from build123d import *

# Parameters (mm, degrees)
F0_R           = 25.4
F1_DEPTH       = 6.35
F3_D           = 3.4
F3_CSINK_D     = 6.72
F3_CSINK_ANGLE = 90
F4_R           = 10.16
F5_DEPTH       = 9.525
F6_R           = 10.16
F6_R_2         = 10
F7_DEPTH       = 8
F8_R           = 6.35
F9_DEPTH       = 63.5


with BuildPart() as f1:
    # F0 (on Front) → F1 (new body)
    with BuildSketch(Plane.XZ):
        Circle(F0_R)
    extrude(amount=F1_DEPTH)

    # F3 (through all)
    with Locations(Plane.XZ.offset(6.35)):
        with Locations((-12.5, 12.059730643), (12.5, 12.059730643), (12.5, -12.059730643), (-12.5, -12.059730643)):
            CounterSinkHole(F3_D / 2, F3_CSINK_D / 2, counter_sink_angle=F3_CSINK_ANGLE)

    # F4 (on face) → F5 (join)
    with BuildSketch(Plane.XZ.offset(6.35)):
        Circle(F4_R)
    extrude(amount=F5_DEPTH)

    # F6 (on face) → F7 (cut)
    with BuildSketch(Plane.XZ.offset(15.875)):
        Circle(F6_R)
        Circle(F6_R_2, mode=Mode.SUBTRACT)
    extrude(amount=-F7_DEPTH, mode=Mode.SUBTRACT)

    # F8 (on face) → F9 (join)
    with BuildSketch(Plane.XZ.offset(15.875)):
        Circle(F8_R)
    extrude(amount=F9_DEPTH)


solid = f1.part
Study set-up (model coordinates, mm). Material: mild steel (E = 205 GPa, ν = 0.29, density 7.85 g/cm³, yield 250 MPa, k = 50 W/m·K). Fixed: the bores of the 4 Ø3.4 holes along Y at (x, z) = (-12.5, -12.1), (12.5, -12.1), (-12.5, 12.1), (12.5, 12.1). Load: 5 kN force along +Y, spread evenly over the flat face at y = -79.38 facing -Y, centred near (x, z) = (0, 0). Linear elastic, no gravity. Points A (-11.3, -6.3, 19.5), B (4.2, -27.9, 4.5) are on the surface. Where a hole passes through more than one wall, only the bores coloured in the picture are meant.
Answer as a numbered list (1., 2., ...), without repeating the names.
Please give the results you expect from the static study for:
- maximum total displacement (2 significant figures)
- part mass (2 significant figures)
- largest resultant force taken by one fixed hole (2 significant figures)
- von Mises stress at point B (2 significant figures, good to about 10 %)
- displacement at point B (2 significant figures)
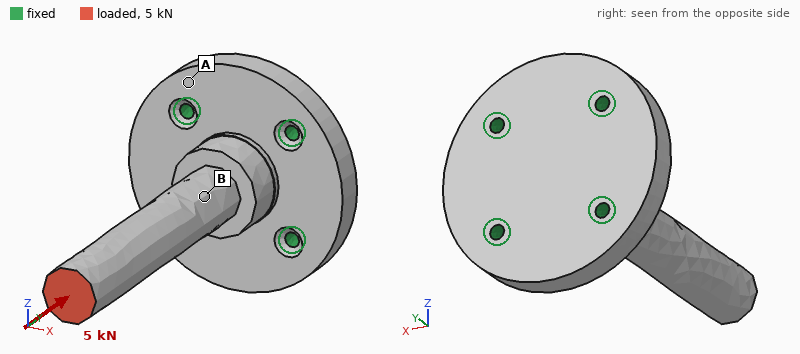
1. 17 µm
2. 190 g
3. 1.4 kN
4. 39 MPa
5. 7.1 µm
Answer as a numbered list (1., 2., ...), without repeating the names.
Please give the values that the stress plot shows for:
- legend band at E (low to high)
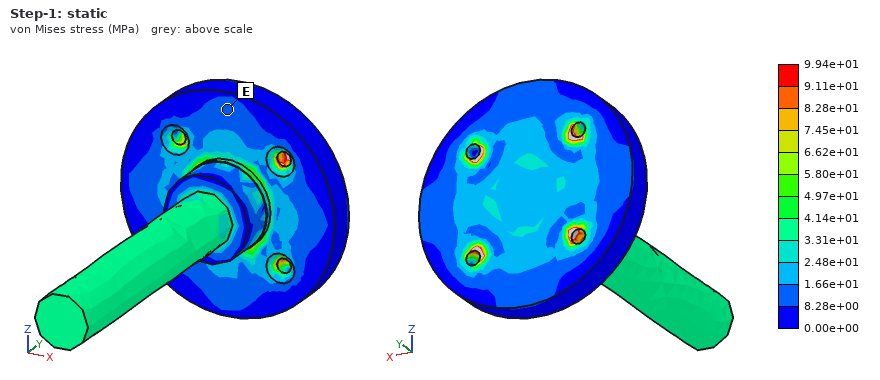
1. 8.28e+00 to 1.66e+01 MPa
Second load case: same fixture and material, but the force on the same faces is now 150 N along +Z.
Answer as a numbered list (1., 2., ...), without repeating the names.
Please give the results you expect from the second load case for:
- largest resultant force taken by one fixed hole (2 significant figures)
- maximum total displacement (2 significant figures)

1. 260 N
2. 64 µm
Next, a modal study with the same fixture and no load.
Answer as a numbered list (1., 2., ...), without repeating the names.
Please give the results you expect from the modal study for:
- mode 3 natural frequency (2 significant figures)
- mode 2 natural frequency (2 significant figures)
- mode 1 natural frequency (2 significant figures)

1. 10 kHz
2. 1900 Hz
3. 1900 Hz
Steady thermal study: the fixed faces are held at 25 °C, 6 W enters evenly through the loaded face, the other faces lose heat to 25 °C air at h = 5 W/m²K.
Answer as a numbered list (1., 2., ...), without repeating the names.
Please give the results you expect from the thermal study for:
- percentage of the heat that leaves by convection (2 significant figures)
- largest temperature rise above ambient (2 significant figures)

1. 8.4 %
2. 65 K
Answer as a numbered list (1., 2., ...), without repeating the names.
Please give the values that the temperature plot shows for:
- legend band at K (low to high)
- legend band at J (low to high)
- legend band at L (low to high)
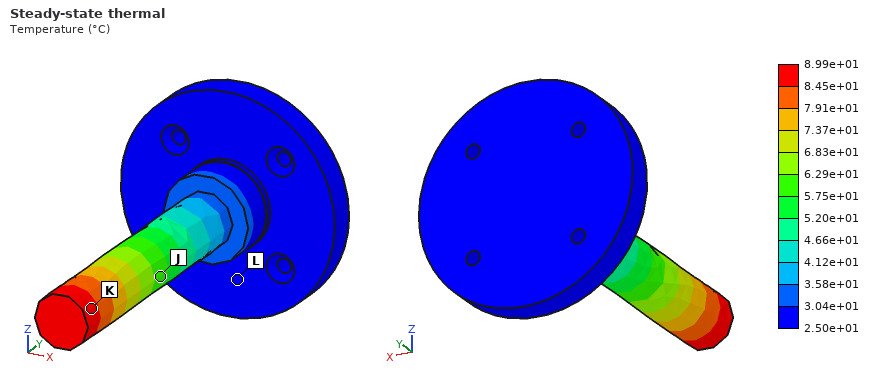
1. 8.45e+01 to 8.99e+01 °C
2. 5.75e+01 to 6.29e+01 °C
3. 2.50e+01 to 3.04e+01 °C
